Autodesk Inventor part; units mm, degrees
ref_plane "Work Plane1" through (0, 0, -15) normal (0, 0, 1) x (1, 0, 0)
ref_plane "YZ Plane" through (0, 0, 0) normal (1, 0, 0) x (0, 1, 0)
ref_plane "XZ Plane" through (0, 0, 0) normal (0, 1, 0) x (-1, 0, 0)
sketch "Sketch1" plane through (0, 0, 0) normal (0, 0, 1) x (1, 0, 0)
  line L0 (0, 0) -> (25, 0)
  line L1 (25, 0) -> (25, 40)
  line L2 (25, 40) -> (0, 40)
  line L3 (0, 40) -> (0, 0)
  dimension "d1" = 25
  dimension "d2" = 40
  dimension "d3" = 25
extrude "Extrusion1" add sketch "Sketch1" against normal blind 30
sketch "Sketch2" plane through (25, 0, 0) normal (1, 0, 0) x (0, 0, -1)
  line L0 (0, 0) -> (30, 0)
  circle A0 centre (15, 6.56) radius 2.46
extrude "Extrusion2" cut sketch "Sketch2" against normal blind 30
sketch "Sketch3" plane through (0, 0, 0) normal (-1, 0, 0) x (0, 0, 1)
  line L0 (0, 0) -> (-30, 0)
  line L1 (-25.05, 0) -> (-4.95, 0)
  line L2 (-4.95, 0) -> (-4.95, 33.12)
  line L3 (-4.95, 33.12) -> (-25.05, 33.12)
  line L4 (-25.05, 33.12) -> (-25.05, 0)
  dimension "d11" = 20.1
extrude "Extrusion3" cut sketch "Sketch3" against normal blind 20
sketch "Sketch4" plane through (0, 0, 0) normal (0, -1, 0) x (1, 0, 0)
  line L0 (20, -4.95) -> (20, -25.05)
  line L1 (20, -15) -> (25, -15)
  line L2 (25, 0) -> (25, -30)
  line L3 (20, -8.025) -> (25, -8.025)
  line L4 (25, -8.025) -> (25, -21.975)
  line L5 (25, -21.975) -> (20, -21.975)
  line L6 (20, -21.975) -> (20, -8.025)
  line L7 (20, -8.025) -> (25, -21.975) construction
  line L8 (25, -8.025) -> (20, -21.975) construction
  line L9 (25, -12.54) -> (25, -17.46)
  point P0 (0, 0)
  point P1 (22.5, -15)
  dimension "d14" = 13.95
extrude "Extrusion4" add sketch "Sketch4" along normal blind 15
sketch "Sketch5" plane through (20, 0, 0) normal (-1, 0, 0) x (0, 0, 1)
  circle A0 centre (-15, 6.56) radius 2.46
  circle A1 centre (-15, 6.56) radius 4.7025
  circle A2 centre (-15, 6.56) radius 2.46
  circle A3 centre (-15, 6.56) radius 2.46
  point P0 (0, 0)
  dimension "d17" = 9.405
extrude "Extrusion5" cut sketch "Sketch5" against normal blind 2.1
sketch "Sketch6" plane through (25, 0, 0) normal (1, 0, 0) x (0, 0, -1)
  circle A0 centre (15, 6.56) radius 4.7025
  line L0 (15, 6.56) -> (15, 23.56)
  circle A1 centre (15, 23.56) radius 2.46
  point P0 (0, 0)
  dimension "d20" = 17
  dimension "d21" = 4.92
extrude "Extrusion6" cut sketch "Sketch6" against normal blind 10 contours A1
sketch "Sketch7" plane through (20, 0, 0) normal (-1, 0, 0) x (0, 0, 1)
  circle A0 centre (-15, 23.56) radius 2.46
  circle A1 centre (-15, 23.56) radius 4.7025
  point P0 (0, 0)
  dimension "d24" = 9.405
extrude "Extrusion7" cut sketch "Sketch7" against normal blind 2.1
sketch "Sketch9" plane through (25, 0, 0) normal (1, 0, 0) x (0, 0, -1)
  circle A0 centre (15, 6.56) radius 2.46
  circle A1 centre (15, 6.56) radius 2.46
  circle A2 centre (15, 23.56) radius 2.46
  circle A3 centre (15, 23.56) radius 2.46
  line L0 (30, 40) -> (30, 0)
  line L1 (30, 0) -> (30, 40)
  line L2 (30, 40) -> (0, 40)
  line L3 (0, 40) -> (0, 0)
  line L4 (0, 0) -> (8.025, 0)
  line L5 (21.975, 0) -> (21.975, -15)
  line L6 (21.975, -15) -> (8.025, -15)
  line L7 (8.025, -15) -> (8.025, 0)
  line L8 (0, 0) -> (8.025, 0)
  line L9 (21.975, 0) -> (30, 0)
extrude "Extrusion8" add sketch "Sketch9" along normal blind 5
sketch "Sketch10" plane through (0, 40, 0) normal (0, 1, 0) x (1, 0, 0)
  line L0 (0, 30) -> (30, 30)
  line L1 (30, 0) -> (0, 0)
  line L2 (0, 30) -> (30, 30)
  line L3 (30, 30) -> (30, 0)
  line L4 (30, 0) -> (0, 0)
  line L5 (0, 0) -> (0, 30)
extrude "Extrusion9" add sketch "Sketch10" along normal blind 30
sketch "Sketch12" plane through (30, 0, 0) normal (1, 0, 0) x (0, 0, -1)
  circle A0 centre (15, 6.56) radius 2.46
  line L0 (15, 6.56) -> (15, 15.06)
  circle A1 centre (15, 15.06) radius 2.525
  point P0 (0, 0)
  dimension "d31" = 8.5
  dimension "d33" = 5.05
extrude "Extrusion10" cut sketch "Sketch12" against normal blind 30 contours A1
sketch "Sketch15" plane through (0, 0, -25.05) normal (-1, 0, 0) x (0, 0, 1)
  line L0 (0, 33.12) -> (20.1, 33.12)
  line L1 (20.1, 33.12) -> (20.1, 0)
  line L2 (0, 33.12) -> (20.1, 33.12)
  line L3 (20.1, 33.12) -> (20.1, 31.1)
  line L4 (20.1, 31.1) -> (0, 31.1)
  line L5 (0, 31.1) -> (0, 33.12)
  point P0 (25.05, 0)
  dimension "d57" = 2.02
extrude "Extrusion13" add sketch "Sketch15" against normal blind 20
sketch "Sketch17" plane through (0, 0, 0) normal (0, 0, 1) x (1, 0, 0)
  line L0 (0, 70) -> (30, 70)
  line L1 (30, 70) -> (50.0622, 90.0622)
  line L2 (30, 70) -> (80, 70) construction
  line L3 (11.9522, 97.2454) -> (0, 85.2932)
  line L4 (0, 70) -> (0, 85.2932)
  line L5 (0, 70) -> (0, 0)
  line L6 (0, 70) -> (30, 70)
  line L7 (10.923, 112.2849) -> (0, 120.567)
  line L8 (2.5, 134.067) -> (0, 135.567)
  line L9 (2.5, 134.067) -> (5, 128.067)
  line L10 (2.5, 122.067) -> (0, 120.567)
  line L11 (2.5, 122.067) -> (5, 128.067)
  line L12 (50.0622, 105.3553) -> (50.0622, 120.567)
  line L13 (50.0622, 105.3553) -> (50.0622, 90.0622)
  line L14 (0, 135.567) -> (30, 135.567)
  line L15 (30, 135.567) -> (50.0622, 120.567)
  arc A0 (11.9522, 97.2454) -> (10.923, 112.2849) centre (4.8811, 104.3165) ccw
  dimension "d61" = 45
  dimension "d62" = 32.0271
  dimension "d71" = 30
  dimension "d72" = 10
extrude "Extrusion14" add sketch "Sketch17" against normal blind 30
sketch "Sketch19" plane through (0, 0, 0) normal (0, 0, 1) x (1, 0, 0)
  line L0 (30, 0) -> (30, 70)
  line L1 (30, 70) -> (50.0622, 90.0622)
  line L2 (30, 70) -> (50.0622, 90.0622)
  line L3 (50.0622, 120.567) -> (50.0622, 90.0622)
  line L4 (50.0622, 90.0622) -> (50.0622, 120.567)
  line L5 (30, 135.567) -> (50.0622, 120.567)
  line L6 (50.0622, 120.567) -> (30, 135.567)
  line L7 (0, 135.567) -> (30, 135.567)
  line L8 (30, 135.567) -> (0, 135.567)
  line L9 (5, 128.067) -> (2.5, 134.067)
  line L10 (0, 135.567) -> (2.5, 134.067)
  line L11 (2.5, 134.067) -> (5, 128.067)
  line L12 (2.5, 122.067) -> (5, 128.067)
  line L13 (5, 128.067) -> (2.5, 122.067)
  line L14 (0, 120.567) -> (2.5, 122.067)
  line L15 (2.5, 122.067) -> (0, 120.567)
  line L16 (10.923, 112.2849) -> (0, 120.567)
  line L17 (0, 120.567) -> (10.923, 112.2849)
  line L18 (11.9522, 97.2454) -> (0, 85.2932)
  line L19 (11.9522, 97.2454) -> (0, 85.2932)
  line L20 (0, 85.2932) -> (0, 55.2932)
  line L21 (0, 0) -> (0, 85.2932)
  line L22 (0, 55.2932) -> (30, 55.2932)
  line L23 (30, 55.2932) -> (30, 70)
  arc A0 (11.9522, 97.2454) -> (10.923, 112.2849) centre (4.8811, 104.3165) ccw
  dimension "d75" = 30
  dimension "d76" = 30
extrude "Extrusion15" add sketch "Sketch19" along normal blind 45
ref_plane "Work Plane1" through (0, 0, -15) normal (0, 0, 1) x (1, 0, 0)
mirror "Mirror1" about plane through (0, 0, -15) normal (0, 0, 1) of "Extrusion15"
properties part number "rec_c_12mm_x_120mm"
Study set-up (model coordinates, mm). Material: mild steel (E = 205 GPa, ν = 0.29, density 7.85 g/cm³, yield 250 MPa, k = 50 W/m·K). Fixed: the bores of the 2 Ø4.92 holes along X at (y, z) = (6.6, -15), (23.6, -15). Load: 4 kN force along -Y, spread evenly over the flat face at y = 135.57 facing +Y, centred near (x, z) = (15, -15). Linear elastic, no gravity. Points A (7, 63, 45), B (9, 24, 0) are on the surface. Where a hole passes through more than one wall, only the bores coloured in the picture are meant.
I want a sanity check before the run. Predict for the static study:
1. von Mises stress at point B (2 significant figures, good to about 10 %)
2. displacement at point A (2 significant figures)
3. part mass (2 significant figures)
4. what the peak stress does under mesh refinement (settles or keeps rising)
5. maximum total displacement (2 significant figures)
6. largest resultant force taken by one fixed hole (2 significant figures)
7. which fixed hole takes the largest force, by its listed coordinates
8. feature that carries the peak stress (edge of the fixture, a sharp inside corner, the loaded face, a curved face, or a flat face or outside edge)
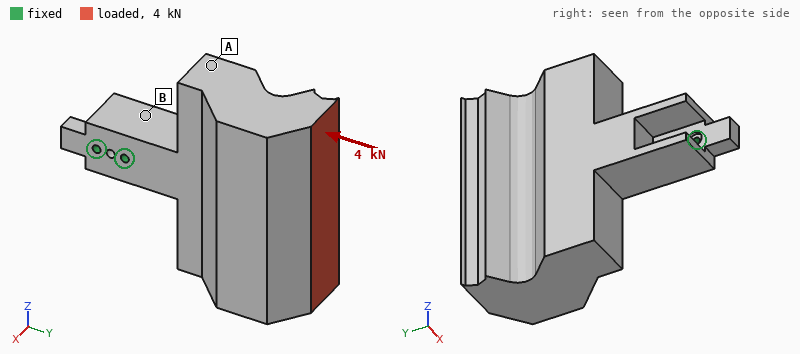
11 MPa
14 µm
3.1 kg
keeps rising
37 µm
3.0 kN
(23.6, -15)
edge of the fixture
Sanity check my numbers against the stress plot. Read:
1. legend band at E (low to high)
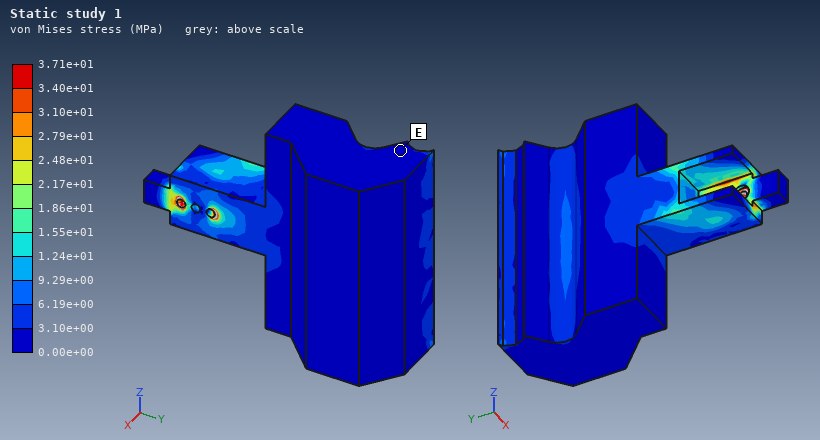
0.00e+00 to 3.10e+00 MPa
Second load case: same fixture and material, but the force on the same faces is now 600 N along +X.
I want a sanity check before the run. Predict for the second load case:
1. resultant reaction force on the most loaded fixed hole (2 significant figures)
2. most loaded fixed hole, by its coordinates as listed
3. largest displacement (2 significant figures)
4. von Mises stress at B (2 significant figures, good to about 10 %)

3.3 kN
(23.6, -15)
71 µm
18 MPa
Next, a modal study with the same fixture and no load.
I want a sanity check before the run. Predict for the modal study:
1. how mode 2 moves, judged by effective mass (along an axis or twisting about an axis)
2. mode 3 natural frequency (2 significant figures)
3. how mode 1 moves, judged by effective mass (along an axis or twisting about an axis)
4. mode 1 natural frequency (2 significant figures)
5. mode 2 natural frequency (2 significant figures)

along Z
600 Hz
along X
410 Hz
430 Hz
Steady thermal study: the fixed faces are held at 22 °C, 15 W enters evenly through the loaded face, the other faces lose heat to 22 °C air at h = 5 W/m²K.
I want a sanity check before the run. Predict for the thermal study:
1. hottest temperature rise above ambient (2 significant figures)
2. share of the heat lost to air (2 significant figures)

25 K
24 %
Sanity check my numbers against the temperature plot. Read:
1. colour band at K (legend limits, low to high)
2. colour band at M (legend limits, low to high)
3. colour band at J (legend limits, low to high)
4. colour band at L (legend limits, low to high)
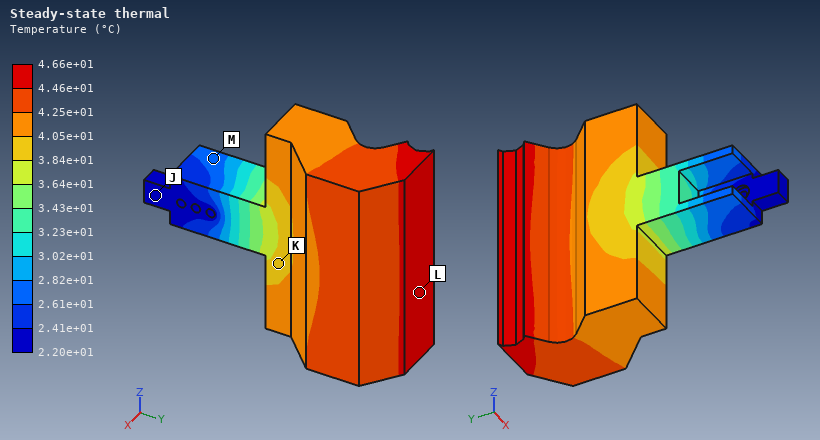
3.84e+01 to 4.05e+01 °C
2.61e+01 to 2.82e+01 °C
2.20e+01 to 2.41e+01 °C
4.46e+01 to 4.66e+01 °C
